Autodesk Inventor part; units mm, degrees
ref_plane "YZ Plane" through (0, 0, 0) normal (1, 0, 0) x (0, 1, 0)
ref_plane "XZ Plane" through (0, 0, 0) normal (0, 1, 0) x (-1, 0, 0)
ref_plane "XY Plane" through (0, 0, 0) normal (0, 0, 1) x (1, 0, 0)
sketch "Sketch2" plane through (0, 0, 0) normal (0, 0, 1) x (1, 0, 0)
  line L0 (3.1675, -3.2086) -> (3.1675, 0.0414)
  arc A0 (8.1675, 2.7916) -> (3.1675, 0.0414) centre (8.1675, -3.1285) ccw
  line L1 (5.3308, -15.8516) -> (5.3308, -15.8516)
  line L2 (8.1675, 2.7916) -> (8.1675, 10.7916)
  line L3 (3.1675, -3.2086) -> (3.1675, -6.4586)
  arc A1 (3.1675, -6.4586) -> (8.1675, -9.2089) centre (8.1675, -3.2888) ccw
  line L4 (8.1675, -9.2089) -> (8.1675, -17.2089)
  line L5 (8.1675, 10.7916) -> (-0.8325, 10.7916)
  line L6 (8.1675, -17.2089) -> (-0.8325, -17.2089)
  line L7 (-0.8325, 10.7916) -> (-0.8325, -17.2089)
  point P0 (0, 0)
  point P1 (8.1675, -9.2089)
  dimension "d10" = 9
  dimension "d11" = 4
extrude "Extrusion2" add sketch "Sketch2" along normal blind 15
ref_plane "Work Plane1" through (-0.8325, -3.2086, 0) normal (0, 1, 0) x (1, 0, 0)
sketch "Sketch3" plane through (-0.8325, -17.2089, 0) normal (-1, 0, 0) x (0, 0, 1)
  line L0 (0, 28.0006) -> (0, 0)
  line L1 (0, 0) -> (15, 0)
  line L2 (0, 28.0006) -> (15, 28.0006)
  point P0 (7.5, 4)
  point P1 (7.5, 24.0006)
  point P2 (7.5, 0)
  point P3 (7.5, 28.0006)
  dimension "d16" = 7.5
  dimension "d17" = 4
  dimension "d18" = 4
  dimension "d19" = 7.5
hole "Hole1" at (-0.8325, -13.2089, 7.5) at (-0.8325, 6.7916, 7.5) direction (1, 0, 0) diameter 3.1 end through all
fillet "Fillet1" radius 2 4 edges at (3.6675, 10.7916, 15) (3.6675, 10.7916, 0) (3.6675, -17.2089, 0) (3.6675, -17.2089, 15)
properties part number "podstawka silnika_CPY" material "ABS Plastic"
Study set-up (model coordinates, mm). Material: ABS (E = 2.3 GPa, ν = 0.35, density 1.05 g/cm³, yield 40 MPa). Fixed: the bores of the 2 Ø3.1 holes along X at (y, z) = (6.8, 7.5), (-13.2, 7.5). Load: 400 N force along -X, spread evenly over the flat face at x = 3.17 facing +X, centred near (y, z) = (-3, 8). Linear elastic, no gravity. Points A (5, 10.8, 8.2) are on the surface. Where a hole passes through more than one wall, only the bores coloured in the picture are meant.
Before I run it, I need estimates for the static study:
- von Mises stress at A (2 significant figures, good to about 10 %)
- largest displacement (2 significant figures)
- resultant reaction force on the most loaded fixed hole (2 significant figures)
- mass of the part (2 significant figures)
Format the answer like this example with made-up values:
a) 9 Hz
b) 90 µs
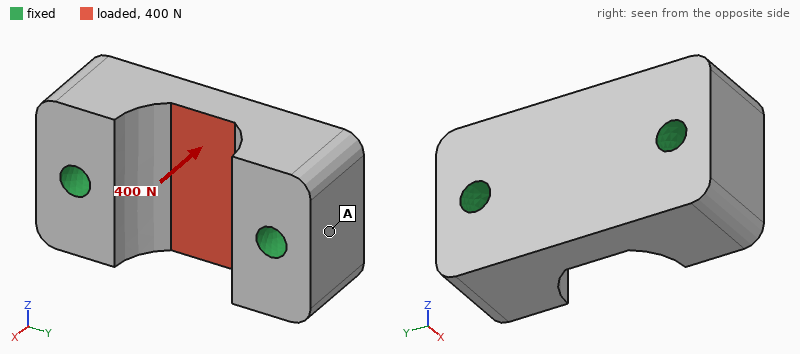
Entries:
a) 2.3 MPa
b) 60 µm
c) 220 N
d) 3.0 g
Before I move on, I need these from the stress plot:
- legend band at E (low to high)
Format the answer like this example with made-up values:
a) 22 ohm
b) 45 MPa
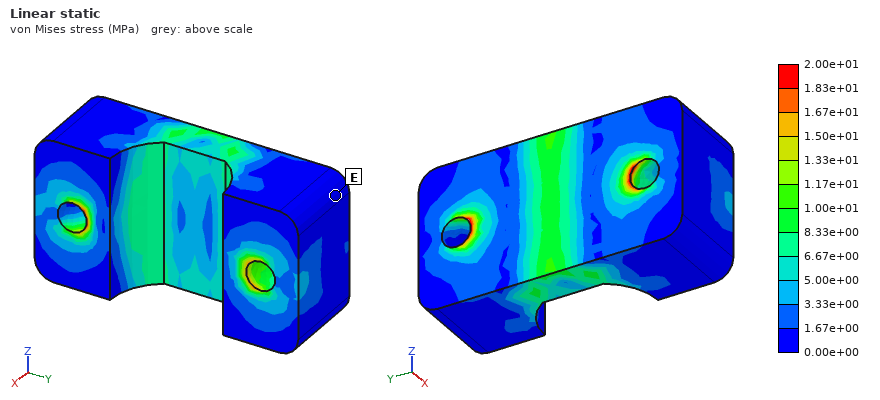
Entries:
a) 0.00e+00 to 1.67e+00 MPa
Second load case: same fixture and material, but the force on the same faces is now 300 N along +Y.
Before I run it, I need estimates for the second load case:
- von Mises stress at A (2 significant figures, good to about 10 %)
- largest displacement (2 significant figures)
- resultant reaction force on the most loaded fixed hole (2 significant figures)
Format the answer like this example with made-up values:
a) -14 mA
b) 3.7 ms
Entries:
a) 1.2 MPa
b) 17 µm
c) 150 N
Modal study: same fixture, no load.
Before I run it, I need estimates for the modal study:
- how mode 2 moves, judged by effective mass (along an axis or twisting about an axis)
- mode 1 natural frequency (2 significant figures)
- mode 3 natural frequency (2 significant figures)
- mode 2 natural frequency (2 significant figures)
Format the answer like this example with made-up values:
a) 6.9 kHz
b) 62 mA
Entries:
a) along X
b) 16 kHz
c) 20 kHz
d) 18 kHz
